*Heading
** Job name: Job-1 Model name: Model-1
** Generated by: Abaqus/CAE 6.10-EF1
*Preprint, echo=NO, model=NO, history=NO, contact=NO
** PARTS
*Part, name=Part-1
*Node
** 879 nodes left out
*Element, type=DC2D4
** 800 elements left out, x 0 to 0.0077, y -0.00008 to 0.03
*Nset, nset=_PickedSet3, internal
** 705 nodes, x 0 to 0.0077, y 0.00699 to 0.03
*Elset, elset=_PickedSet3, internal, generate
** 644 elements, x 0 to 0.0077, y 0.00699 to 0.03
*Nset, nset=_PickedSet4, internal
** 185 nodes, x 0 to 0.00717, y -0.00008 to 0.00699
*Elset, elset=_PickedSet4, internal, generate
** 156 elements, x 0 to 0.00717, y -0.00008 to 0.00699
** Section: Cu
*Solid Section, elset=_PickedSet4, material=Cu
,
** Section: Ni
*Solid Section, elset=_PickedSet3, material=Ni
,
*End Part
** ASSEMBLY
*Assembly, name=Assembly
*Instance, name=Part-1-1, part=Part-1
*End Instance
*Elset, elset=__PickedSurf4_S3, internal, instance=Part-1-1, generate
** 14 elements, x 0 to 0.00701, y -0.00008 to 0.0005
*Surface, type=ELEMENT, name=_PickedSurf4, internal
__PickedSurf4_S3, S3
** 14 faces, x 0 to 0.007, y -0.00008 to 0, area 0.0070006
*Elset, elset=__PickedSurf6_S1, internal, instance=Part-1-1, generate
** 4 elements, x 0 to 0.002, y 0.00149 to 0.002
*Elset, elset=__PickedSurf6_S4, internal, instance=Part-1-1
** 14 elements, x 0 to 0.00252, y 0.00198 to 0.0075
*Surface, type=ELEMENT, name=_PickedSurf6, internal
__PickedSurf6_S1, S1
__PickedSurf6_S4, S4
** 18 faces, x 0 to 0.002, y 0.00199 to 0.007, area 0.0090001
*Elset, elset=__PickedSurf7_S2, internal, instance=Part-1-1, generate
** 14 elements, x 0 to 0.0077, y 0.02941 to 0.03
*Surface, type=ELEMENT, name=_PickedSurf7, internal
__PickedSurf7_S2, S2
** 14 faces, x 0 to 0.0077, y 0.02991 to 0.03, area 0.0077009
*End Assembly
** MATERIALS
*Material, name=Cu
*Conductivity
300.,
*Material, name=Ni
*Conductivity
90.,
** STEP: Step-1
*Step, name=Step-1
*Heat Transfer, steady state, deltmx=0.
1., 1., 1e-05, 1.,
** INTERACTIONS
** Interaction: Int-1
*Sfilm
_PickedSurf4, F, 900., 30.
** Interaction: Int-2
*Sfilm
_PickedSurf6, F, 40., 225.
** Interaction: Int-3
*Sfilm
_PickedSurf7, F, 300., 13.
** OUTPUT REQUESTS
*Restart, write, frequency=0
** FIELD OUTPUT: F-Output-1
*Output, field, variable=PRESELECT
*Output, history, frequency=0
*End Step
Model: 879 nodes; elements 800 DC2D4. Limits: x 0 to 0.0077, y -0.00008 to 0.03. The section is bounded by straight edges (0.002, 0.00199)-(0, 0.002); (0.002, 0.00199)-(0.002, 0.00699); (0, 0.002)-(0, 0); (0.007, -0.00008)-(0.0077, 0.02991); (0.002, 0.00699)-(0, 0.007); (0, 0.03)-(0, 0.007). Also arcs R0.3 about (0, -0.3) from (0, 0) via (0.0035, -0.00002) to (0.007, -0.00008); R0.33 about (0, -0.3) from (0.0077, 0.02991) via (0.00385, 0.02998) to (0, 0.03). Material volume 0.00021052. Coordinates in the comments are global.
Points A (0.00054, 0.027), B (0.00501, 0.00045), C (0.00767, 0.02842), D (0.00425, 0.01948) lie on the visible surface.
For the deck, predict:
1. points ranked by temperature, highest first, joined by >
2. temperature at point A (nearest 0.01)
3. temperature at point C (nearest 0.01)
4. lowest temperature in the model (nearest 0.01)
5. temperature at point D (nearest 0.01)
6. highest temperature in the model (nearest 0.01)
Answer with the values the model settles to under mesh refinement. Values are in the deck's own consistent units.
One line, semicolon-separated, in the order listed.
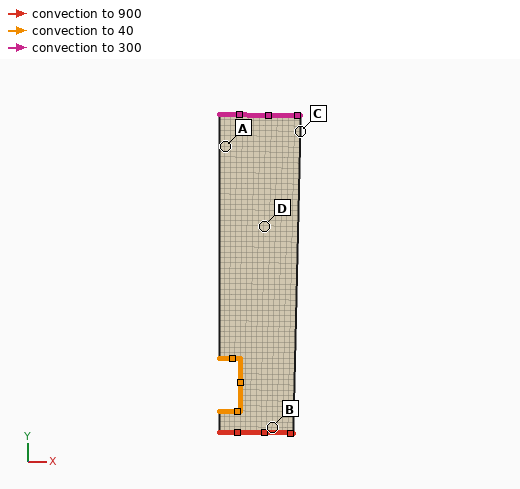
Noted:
C > A > B > D; 128.88; 128.92; 128.01; 128.69; 128.96
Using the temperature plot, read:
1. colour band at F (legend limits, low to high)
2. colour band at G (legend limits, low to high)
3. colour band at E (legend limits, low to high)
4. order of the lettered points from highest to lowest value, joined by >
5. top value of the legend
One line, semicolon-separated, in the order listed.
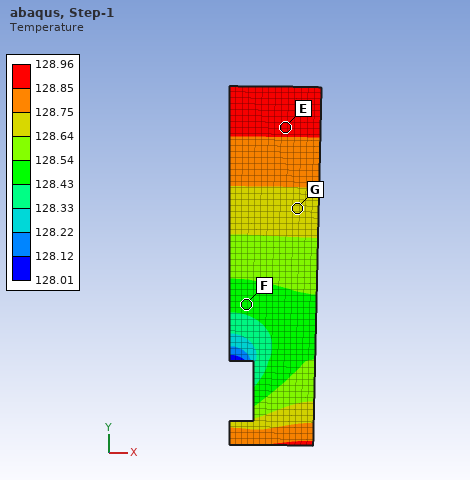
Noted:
128.43 to 128.54; 128.64 to 128.75; 128.85 to 128.96; E > G > F; 128.96
